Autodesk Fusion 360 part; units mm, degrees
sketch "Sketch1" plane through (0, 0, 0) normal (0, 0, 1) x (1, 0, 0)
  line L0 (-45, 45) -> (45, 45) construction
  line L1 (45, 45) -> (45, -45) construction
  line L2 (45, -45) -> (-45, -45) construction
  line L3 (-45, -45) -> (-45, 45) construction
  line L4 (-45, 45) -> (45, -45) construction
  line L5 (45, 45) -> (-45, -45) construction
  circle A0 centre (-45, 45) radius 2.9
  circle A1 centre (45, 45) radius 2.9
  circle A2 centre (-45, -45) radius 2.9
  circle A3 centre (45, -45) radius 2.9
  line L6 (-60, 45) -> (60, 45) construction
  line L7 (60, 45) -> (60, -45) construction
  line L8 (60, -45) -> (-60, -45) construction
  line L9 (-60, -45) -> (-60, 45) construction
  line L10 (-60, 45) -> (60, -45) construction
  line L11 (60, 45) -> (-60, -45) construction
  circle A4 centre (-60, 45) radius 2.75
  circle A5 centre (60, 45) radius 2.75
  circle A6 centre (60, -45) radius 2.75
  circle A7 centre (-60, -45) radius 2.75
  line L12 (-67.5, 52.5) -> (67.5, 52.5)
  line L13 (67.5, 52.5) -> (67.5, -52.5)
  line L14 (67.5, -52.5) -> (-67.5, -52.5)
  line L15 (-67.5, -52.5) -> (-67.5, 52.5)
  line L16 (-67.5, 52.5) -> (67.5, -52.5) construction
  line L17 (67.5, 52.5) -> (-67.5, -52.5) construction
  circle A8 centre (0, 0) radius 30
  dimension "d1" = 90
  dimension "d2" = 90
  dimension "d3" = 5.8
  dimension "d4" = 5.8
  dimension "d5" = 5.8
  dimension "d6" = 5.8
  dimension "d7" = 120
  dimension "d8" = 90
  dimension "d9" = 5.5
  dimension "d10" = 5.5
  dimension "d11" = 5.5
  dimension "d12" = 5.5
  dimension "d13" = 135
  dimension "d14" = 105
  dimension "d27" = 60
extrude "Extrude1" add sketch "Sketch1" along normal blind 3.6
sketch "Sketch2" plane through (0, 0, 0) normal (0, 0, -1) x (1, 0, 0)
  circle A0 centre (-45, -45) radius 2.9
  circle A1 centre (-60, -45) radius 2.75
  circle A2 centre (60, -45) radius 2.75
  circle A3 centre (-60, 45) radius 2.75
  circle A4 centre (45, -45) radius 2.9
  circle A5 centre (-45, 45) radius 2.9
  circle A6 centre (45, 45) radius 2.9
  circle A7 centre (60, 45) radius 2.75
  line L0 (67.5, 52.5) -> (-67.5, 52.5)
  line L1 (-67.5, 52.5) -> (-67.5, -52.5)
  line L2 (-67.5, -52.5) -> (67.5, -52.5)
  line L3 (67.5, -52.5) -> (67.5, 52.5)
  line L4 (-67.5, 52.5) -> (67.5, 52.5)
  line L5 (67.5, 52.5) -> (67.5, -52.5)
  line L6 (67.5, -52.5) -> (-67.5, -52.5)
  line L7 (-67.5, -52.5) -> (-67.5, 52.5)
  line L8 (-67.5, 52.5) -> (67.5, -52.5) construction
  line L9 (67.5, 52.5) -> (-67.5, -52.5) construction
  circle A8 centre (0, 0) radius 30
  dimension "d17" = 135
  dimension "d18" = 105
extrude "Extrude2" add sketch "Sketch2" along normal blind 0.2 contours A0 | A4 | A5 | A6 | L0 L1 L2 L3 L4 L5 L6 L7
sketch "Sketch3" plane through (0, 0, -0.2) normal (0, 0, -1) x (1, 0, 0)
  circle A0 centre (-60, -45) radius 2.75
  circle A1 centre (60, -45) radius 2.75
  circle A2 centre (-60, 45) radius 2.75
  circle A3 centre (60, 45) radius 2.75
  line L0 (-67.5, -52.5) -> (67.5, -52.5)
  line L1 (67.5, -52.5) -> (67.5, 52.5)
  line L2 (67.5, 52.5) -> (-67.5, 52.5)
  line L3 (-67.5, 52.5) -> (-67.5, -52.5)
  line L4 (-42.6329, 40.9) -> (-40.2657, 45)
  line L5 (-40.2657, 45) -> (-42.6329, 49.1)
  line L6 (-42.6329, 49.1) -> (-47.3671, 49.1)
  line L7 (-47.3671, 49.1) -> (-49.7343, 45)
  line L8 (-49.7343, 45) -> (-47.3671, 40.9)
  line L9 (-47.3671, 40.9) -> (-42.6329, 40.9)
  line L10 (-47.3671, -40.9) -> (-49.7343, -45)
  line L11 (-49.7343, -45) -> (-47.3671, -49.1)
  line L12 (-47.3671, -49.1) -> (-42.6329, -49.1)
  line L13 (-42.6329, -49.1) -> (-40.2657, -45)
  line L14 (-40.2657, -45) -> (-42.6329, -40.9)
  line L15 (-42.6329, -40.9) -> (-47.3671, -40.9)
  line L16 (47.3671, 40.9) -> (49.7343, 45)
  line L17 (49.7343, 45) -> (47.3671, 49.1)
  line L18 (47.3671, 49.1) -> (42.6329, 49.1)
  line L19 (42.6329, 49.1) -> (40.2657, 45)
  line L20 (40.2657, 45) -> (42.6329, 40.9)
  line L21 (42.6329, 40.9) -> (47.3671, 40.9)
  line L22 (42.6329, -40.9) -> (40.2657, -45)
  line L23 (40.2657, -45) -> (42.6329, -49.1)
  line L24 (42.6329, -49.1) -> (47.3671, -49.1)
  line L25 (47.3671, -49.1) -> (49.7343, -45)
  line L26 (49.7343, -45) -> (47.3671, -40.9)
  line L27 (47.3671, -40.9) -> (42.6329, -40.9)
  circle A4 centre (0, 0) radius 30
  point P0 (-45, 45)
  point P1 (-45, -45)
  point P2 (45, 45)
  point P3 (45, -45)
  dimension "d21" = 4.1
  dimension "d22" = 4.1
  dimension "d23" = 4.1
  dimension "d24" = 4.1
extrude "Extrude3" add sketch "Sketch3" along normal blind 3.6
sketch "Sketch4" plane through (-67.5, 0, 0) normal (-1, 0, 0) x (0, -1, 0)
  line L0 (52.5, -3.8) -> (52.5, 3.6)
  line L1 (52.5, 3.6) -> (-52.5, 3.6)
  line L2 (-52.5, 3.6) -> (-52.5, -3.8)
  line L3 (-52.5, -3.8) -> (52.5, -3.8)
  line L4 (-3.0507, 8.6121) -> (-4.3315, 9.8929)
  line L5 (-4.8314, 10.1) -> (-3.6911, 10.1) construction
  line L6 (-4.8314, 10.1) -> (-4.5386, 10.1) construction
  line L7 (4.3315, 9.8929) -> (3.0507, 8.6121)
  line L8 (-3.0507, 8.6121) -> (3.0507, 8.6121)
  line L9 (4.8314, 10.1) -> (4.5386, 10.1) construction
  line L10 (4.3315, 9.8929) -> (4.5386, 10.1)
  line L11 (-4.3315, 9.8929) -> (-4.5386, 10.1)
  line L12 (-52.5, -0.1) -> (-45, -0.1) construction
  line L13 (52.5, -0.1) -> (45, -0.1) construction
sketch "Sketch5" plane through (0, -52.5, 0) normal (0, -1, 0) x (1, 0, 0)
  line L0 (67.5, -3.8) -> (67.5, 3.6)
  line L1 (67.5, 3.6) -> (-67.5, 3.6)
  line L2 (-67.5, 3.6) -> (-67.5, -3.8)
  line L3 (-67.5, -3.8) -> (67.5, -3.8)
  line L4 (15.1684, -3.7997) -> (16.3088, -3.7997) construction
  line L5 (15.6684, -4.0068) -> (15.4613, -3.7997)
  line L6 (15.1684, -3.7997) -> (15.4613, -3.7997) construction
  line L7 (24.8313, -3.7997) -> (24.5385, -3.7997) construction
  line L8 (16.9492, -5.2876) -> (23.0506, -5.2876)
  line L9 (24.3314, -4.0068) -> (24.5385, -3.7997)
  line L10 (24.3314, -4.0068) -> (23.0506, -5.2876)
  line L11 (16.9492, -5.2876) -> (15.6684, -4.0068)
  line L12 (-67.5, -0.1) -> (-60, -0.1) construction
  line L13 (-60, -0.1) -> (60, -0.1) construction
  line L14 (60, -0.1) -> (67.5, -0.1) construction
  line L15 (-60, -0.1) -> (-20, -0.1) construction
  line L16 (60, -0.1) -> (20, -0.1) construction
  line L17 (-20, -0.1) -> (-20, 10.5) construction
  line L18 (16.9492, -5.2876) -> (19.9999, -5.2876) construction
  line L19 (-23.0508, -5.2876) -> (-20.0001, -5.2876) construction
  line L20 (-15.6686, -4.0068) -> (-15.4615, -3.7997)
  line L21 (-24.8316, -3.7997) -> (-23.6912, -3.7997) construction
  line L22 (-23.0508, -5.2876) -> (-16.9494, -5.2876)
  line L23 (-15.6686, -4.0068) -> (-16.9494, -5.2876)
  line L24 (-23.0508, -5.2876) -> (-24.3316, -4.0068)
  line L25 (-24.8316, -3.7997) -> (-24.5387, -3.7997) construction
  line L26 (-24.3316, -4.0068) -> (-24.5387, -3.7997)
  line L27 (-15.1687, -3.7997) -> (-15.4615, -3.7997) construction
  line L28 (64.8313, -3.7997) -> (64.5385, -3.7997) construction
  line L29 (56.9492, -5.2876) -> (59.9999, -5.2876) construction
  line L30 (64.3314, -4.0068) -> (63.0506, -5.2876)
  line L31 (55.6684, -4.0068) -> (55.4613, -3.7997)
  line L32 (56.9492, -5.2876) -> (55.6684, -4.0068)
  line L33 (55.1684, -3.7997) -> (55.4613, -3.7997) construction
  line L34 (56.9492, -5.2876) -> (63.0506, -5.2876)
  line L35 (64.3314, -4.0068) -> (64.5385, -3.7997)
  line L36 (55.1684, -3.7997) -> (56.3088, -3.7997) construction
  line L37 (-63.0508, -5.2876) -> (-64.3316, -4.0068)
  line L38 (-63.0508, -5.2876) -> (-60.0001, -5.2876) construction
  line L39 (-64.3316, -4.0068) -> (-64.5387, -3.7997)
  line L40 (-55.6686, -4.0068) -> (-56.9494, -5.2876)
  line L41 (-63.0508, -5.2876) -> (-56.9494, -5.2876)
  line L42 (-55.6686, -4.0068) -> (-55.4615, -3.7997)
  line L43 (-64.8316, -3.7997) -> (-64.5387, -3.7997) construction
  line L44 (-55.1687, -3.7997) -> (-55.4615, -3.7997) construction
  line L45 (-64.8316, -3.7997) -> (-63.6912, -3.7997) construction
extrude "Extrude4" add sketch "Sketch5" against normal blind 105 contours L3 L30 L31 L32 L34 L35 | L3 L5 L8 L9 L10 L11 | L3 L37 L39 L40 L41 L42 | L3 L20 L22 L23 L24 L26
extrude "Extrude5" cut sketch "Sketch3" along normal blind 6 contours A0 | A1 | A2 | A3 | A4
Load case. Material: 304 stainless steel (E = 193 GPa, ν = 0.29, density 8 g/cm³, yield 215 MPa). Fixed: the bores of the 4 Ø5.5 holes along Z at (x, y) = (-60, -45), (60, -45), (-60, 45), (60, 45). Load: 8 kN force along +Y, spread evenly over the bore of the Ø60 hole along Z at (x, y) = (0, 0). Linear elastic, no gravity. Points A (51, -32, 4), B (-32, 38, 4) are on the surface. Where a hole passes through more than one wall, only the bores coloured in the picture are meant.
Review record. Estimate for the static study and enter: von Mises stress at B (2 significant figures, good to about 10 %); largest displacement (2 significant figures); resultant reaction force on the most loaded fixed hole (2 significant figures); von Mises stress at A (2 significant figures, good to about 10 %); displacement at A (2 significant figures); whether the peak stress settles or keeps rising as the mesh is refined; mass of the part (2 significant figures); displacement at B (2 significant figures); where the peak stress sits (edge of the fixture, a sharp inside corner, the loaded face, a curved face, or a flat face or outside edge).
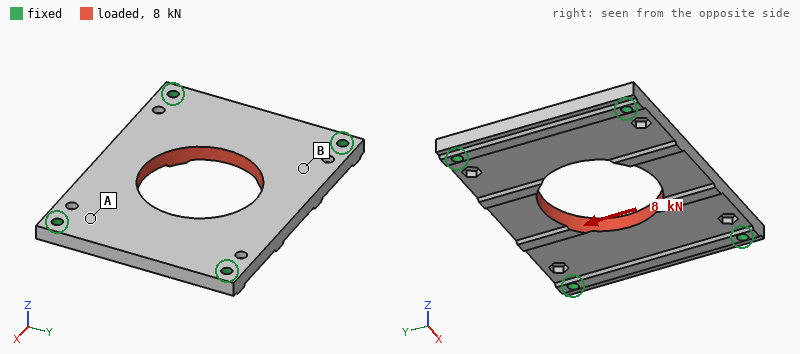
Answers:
6.4 MPa
6.5 µm
2.2 kN
11 MPa
1.4 µm
keeps rising
690 g
3.5 µm
edge of the fixture
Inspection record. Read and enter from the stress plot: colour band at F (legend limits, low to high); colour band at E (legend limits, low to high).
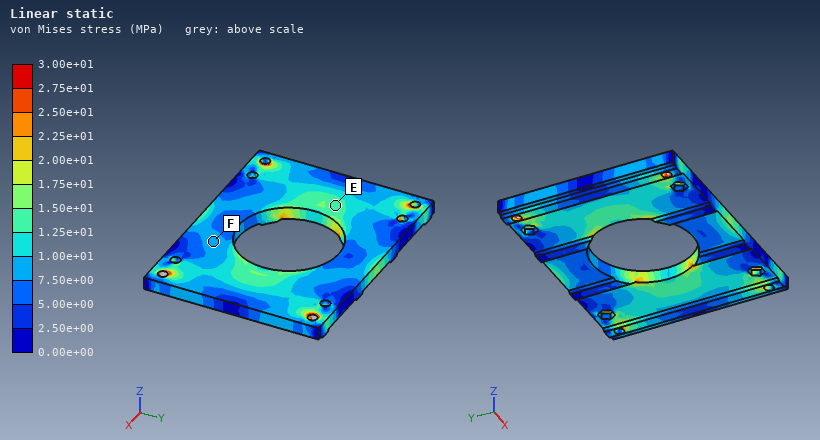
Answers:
7.50e+00 to 1.00e+01 MPa
1.25e+01 to 1.50e+01 MPa
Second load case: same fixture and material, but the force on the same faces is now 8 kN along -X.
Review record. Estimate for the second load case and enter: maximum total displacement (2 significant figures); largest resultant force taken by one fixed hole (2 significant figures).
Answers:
3.9 µm
2.2 kN
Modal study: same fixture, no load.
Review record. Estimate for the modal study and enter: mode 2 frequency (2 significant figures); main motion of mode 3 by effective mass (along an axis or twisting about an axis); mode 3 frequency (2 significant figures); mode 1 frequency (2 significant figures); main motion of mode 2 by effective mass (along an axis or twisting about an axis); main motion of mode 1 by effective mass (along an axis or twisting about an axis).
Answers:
2900 Hz
twisting about Y
4100 Hz
2200 Hz
twisting about X
along Z
